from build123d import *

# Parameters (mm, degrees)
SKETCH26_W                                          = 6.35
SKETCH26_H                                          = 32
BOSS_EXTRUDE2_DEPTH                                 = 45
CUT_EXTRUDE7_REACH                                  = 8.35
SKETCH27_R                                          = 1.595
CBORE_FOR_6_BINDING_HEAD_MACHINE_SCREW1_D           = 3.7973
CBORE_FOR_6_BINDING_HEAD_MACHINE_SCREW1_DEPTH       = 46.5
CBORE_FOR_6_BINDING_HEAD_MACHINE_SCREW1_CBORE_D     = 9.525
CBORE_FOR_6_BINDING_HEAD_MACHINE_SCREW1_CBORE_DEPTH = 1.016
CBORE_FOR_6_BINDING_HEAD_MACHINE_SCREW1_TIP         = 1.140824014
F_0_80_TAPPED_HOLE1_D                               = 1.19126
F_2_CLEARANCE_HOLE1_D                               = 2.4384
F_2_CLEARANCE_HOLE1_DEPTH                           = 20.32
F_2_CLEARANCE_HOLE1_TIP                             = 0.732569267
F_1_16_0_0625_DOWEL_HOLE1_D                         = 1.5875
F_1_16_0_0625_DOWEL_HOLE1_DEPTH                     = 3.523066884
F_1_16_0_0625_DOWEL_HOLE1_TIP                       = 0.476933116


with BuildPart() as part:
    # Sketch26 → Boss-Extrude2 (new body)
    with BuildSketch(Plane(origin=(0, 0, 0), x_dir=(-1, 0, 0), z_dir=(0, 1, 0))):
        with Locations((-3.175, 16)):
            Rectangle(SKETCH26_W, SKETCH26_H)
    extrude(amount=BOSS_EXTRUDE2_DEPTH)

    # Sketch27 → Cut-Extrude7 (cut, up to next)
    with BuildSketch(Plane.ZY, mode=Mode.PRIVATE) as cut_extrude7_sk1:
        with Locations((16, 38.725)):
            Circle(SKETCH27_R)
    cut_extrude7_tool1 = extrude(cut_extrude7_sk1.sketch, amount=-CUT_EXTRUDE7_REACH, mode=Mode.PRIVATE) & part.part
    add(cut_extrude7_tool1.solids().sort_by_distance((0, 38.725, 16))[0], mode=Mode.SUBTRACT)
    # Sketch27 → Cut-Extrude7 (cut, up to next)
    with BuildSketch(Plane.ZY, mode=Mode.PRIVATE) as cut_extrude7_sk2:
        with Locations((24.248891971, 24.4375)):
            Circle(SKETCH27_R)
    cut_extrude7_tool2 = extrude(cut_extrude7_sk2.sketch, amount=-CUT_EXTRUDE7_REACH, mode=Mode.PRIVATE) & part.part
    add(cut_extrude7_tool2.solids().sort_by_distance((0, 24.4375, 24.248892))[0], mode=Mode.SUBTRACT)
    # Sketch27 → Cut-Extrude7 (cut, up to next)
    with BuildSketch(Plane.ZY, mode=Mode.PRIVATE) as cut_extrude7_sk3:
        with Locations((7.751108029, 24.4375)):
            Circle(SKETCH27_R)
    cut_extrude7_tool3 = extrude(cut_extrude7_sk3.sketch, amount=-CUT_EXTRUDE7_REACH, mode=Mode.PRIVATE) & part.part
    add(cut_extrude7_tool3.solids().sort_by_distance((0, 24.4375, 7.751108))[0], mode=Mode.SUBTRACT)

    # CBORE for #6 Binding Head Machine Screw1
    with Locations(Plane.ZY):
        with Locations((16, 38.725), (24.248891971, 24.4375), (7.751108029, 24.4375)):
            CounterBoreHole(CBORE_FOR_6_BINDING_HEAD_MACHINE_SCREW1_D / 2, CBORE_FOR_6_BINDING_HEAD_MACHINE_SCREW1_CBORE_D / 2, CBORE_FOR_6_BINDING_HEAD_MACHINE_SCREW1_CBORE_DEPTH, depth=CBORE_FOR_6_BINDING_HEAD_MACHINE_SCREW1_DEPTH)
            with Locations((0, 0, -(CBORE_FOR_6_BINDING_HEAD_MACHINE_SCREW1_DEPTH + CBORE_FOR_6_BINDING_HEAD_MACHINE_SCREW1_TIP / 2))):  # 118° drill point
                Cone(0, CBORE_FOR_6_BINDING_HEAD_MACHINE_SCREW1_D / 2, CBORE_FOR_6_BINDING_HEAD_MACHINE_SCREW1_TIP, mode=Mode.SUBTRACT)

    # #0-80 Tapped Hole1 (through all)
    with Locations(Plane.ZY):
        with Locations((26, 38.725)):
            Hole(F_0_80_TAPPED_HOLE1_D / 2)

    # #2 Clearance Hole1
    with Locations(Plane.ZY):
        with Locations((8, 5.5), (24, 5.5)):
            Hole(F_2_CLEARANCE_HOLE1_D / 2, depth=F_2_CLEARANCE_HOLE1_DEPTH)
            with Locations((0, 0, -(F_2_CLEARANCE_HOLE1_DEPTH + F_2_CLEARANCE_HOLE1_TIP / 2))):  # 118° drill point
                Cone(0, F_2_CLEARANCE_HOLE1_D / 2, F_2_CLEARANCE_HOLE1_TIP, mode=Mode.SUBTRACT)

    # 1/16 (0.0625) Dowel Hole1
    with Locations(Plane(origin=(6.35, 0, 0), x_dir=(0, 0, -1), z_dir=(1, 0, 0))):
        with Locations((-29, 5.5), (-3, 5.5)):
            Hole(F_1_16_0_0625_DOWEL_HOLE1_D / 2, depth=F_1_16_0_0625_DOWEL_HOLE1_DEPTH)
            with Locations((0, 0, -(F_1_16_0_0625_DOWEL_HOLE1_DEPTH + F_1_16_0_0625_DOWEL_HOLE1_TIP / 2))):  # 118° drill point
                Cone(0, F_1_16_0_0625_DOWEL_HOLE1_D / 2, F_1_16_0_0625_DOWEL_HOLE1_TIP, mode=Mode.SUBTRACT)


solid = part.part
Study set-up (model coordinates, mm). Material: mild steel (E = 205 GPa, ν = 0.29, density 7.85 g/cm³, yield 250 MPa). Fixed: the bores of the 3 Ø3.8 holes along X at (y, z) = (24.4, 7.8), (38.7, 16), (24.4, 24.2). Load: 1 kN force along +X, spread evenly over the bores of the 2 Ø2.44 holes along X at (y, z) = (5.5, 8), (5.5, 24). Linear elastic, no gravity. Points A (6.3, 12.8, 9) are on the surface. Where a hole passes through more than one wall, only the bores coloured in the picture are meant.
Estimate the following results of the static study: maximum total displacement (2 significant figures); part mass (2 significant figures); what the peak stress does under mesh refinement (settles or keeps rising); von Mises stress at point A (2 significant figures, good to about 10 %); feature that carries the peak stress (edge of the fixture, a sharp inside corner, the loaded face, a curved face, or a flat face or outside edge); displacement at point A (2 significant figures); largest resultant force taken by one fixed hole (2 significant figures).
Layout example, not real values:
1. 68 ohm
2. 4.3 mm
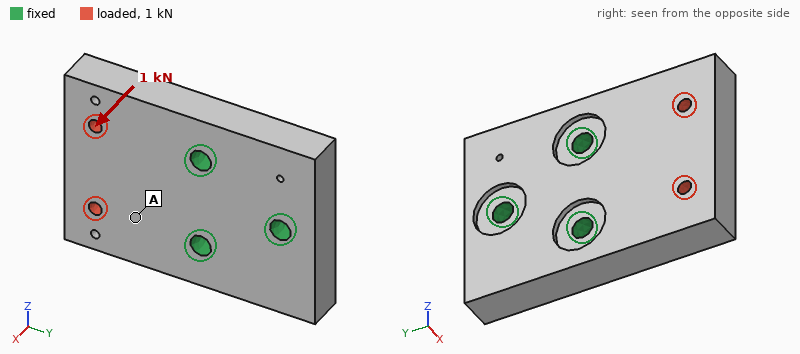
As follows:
1. 31 µm
2. 68 g
3. keeps rising
4. 33 MPa
5. edge of the fixture
6. 11 µm
7. 660 N
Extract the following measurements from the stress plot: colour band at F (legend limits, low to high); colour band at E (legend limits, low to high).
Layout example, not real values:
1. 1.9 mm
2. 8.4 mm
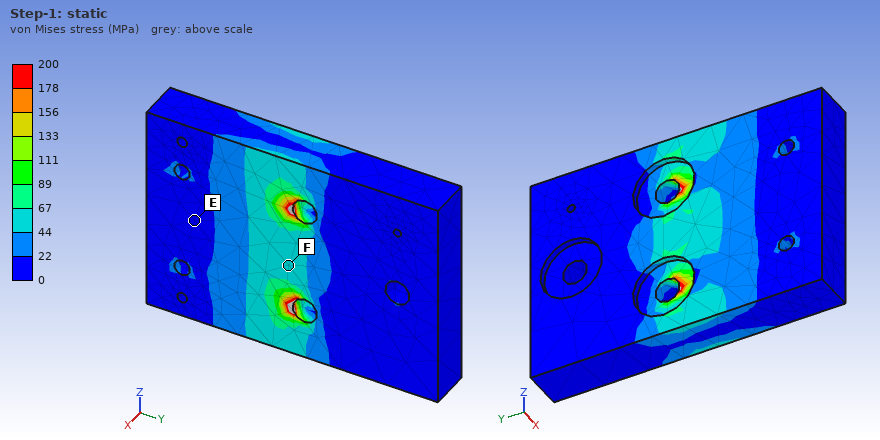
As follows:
1. 44 to 67 MPa
2. 0 to 22 MPa
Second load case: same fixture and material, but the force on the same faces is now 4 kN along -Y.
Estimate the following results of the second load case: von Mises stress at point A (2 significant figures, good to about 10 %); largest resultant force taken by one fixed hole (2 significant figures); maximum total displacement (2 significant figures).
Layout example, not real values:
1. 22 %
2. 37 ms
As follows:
1. 27 MPa
2. 1.8 kN
3. 3.4 µm
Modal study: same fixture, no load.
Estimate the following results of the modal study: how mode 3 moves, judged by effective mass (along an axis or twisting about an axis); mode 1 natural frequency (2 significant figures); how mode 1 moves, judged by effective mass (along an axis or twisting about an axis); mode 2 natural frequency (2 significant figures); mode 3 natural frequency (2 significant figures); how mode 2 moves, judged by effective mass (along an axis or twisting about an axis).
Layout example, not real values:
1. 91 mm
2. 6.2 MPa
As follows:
1. along Z
2. 7600 Hz
3. along X
4. 14 kHz
5. 21 kHz
6. twisting about Y
